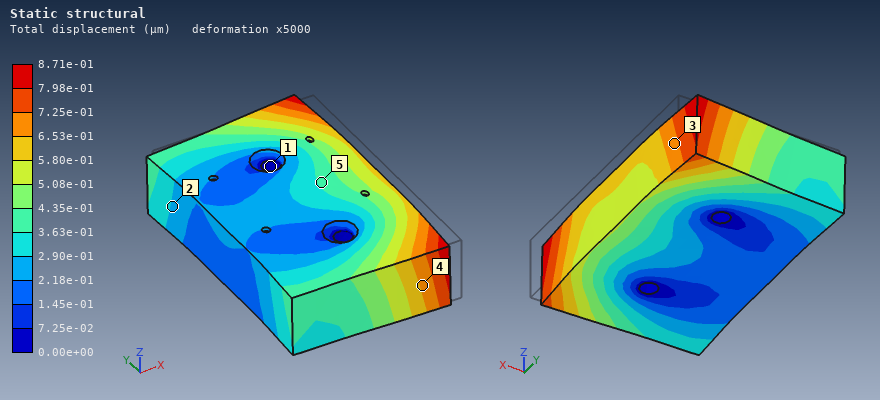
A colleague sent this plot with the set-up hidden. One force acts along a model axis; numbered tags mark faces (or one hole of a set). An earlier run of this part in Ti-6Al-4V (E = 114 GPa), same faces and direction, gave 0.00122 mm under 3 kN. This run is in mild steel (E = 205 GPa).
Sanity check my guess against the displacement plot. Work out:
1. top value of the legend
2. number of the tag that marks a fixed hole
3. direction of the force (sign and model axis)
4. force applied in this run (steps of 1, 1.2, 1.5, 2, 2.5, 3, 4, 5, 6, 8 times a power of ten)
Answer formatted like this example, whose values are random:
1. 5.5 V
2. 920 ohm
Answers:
1. 8.71e-01 µm
2. 1
3. -X
4. 4 kN
